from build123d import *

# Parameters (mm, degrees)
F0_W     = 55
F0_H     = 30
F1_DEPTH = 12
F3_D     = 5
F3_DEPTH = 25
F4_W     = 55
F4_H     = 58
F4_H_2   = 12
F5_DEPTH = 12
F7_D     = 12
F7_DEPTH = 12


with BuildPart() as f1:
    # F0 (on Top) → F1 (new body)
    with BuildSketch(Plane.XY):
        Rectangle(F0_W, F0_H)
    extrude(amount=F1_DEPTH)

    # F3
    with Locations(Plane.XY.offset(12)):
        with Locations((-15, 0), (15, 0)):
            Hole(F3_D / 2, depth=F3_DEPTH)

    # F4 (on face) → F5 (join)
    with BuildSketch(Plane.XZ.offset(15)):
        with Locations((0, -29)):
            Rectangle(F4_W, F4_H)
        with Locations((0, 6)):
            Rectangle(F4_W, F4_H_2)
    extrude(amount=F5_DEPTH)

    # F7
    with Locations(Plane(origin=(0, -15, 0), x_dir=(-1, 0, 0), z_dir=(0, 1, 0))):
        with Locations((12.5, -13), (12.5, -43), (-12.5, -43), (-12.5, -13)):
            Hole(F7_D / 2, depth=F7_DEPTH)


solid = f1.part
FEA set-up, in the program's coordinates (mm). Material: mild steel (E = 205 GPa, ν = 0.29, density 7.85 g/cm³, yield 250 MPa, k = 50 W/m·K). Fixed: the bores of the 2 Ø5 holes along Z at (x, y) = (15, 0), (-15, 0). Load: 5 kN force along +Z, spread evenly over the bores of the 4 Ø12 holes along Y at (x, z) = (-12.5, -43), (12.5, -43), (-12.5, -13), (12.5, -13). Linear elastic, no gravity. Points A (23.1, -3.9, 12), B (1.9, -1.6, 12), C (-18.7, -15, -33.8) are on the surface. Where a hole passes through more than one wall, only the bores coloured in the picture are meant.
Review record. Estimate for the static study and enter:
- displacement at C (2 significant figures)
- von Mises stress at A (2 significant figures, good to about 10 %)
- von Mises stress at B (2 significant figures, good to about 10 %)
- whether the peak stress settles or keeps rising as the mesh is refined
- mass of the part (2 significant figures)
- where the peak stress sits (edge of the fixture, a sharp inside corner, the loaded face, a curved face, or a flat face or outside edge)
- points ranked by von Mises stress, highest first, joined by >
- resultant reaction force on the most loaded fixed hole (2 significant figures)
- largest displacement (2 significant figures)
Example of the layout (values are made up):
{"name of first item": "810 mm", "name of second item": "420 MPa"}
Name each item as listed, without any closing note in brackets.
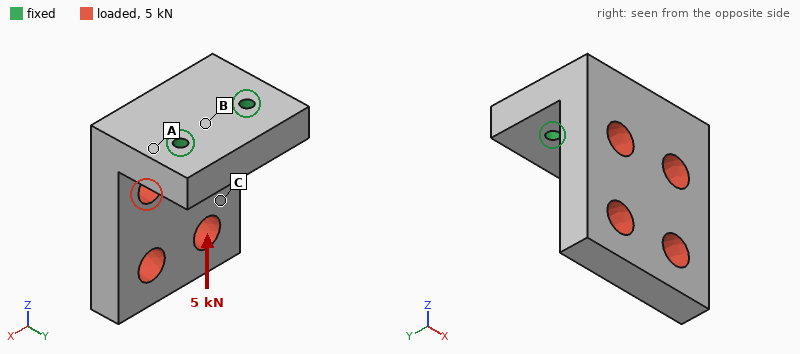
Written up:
{"displacement at C": "36 µm", "von Mises stress at A": "43 MPa", "von Mises stress at B": "30 MPa", "whether the peak stress settles or keeps rising as the mesh is refined": "keeps rising", "mass of the part": "470 g", "where the peak stress sits": "edge of the fixture", "points ranked by von Mises stress, highest first, joined by >": "A > B > C", "resultant reaction force on the most loaded fixed hole": "2.5 kN", "largest displacement": "59 µm"}
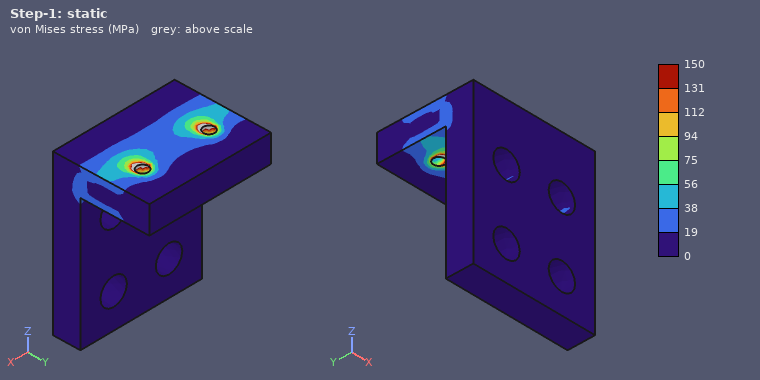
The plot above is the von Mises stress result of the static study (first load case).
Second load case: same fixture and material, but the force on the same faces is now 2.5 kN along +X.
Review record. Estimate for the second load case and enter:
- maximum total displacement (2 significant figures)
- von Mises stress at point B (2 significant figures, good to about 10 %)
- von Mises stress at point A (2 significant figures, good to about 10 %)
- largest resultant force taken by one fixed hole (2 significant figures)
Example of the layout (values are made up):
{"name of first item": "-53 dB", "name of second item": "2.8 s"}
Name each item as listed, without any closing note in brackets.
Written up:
{"maximum total displacement": "31 µm", "von Mises stress at point B": "11 MPa", "von Mises stress at point A": "26 MPa", "largest resultant force taken by one fixed hole": "3.0 kN"}
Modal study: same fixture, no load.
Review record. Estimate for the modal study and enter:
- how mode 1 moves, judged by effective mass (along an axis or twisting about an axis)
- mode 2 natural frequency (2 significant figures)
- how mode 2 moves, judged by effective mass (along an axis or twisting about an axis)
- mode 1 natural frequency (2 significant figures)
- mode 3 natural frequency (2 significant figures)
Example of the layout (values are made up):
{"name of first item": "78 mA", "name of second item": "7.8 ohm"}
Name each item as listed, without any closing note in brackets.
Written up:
{"how mode 1 moves, judged by effective mass": "along Y", "mode 2 natural frequency": "3200 Hz", "how mode 2 moves, judged by effective mass": "along X", "mode 1 natural frequency": "1600 Hz", "mode 3 natural frequency": "5200 Hz"}
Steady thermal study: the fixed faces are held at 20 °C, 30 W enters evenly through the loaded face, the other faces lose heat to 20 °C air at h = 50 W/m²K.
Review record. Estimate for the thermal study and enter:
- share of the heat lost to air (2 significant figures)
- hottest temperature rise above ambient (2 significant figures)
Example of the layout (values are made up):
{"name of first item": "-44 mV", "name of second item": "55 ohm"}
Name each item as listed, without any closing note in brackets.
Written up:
{"share of the heat lost to air": "40 %", "hottest temperature rise above ambient": "35 K"}
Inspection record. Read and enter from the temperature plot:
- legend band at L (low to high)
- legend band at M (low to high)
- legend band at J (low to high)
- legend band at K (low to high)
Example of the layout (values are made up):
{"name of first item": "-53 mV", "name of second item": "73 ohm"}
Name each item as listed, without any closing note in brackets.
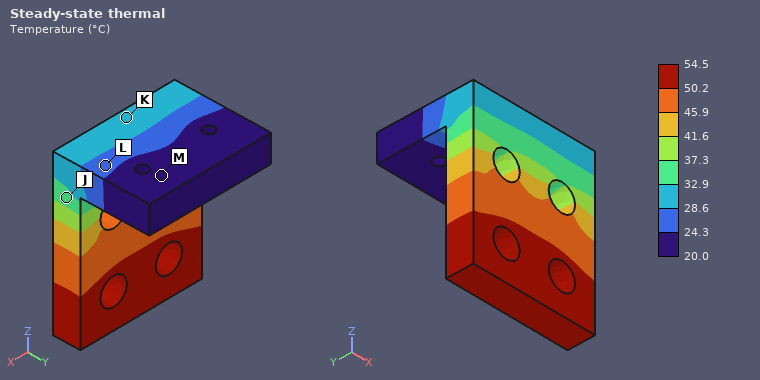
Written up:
{"legend band at L": "24.3 to 28.6 °C", "legend band at M": "20.0 to 24.3 °C", "legend band at J": "32.9 to 37.3 °C", "legend band at K": "28.6 to 32.9 °C"}
